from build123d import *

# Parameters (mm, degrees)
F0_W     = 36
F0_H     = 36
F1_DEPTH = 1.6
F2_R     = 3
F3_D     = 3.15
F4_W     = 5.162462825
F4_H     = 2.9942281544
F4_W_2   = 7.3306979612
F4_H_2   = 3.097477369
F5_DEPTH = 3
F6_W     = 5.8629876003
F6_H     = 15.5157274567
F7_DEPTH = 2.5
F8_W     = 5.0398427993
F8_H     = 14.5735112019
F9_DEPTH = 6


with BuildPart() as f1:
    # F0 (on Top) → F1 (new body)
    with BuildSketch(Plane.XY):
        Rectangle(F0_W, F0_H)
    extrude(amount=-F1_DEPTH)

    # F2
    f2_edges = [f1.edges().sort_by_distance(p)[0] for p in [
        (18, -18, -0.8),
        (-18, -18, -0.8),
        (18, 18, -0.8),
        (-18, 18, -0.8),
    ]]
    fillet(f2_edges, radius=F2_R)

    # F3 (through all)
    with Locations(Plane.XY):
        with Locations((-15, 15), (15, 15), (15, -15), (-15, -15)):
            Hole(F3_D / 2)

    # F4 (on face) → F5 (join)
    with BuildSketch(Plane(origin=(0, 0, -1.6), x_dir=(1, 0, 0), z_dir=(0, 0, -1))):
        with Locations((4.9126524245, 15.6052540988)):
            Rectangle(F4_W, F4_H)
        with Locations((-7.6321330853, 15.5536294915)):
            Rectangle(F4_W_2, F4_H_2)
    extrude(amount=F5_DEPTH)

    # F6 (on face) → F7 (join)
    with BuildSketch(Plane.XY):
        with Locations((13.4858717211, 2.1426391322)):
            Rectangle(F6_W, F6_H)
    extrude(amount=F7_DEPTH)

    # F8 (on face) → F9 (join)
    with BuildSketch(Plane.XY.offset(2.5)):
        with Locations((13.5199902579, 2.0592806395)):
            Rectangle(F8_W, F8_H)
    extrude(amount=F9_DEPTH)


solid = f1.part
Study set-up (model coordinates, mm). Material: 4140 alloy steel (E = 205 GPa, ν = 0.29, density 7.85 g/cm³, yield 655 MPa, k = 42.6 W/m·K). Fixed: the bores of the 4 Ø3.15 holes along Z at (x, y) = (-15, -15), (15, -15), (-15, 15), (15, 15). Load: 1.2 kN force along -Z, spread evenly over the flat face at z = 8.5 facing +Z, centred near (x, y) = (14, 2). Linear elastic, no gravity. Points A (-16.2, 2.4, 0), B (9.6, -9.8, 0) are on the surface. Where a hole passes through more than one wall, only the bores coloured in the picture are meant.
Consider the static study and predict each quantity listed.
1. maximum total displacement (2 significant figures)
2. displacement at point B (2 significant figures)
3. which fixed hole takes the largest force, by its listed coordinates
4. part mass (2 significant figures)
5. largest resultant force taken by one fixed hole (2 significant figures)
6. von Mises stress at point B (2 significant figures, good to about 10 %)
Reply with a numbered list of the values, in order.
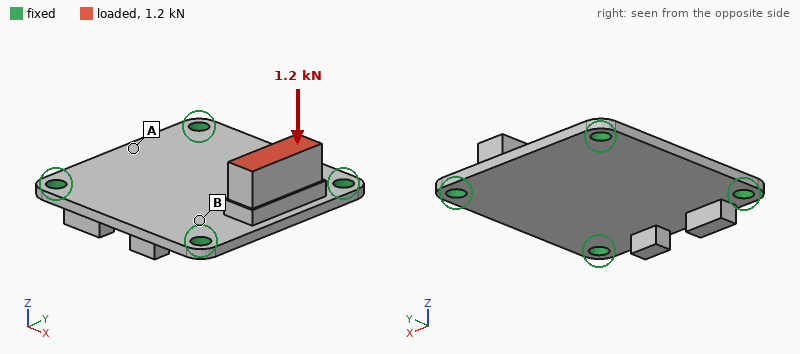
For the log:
1. 51 µm
2. 25 µm
3. (15, 15)
4. 22 g
5. 730 N
6. 120 MPa
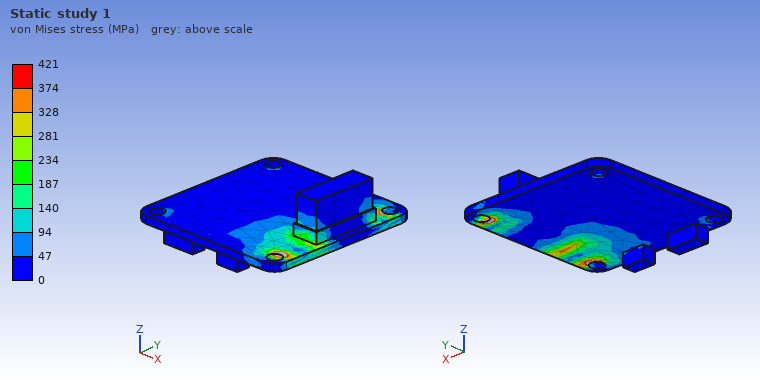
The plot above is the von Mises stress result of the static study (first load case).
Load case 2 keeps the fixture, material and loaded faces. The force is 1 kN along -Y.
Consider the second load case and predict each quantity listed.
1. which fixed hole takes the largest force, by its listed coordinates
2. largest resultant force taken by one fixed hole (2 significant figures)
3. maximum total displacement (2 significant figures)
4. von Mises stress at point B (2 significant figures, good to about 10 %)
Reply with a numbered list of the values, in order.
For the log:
1. (15, 15)
2. 630 N
3. 43 µm
4. 100 MPa
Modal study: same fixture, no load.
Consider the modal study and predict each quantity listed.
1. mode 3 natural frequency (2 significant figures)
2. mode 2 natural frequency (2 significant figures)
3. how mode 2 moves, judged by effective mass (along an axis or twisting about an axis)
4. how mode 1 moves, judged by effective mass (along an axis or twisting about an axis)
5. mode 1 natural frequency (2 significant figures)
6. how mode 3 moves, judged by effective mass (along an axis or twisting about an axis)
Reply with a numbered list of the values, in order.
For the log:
1. 11 kHz
2. 9500 Hz
3. along Z
4. along Z
5. 6500 Hz
6. twisting about X
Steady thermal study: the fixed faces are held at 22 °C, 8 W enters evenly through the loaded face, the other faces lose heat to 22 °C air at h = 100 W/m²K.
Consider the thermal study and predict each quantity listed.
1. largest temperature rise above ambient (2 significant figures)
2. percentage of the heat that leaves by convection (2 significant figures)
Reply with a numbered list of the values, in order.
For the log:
1. 46 K
2. 42 %
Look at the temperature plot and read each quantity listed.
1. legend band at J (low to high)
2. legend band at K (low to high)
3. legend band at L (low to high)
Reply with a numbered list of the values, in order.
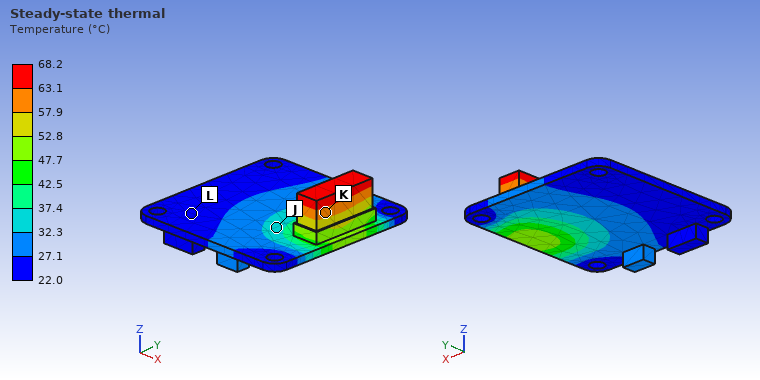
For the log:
1. 32.3 to 37.4 °C
2. 57.9 to 63.1 °C
3. 22.0 to 27.1 °C
